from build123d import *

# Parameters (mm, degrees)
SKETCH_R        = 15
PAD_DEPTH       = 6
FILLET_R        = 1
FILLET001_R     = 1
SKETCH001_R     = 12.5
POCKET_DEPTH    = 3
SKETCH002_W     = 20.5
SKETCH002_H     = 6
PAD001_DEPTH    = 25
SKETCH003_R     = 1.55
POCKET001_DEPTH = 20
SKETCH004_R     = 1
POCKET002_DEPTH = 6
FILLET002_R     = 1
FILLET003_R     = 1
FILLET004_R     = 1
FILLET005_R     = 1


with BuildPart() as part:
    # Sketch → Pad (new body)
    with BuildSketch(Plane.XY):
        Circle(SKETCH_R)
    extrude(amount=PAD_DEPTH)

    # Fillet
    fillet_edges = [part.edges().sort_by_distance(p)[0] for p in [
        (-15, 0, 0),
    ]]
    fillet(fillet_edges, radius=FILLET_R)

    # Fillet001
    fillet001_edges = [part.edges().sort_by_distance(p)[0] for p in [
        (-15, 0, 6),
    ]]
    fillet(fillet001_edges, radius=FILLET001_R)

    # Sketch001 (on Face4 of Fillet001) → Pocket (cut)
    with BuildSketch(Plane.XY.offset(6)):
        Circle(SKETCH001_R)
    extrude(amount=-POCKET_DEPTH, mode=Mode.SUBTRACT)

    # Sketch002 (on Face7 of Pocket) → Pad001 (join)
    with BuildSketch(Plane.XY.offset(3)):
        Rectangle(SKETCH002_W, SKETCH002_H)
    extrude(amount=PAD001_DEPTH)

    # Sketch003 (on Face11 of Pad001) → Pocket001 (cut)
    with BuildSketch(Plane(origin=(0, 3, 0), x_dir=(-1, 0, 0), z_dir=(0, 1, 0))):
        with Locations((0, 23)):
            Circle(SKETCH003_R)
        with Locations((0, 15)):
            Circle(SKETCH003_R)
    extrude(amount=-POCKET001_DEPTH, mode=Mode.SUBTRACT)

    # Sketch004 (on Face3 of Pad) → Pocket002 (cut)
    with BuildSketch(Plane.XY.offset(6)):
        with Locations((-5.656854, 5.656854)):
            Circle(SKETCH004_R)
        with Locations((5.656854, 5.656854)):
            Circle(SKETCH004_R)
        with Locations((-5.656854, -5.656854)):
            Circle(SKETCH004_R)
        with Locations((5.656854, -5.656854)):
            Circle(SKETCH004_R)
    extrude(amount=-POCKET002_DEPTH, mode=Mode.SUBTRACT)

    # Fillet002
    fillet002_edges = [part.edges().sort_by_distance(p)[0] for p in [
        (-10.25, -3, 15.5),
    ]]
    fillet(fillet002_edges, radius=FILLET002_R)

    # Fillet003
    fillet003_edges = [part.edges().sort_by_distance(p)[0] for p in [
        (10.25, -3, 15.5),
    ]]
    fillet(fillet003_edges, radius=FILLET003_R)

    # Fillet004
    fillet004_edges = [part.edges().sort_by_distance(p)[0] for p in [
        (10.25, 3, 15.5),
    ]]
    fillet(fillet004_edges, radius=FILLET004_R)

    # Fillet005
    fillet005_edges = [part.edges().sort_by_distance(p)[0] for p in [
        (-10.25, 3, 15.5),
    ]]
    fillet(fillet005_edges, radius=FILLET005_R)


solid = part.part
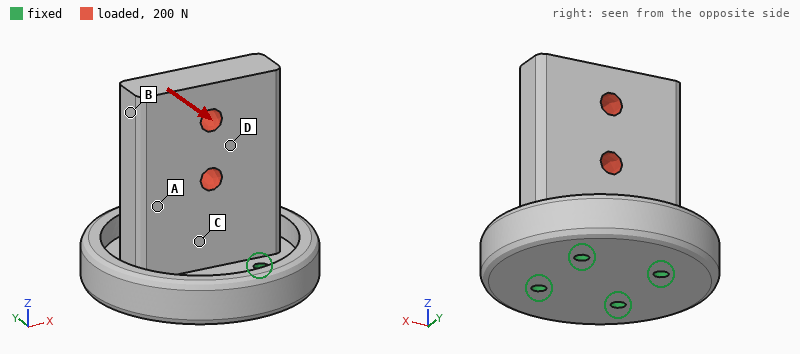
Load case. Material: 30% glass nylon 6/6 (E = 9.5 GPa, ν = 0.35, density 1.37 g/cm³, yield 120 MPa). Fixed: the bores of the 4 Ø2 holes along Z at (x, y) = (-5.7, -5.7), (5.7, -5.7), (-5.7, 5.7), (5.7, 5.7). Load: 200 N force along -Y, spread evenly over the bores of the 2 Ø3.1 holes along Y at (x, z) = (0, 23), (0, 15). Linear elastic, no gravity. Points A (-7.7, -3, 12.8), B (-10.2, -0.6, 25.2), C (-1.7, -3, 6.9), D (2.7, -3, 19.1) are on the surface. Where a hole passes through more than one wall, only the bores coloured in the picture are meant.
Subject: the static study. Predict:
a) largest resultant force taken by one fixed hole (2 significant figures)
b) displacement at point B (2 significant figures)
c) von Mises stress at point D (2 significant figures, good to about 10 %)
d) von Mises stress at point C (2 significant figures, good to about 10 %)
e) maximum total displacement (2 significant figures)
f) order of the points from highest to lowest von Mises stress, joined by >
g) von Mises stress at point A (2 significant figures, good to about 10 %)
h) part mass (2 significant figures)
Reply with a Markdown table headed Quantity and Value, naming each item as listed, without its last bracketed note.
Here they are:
| Quantity | Value |
|---|---|
| largest resultant force taken by one fixed hole | 180 N |
| displacement at point B | 0.20 mm |
| von Mises stress at point D | 6.0 MPa |
| von Mises stress at point C | 18 MPa |
| maximum total displacement | 0.24 mm |
| order of the points from highest to lowest von Mises stress, joined by > | C > A > D > B |
| von Mises stress at point A | 11 MPa |
| part mass | 7.7 g |
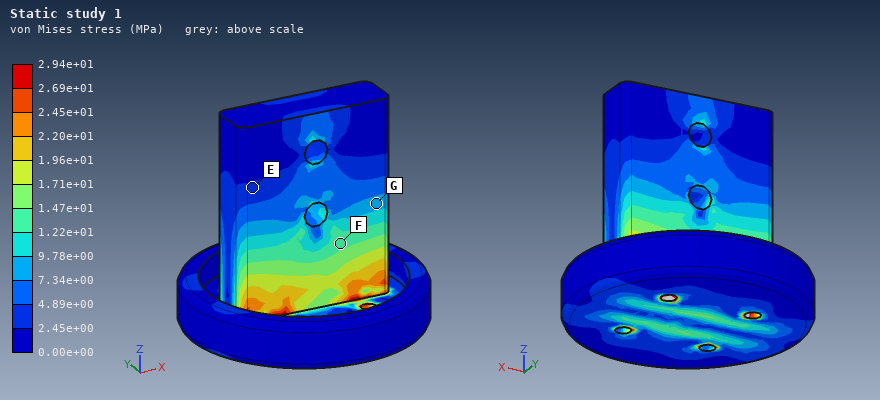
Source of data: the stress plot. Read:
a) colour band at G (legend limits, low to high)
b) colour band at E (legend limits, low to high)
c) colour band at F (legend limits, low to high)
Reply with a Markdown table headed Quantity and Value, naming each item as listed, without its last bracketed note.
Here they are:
| Quantity | Value |
|---|---|
| colour band at G | 7.34e+00 to 9.78e+00 MPa |
| colour band at E | 2.45e+00 to 4.89e+00 MPa |
| colour band at F | 1.22e+01 to 1.47e+01 MPa |
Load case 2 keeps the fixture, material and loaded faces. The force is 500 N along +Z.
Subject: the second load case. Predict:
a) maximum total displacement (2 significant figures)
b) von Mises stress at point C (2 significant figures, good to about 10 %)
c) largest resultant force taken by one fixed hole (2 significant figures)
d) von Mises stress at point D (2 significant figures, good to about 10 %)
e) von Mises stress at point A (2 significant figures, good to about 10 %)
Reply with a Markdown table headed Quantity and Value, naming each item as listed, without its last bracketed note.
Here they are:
| Quantity | Value |
|---|---|
| maximum total displacement | 19 µm |
| von Mises stress at point C | 4.4 MPa |
| largest resultant force taken by one fixed hole | 130 N |
| von Mises stress at point D | 5.1 MPa |
| von Mises stress at point A | 3.1 MPa |
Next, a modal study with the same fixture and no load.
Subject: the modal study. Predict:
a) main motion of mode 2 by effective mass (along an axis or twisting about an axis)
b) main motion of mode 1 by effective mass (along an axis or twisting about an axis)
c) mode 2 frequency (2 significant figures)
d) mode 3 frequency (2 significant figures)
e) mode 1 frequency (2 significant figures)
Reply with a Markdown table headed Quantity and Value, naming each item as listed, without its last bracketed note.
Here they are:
| Quantity | Value |
|---|---|
| main motion of mode 2 by effective mass | along X |
| main motion of mode 1 by effective mass | along Y |
| mode 2 frequency | 5900 Hz |
| mode 3 frequency | 8500 Hz |
| mode 1 frequency | 3300 Hz |
